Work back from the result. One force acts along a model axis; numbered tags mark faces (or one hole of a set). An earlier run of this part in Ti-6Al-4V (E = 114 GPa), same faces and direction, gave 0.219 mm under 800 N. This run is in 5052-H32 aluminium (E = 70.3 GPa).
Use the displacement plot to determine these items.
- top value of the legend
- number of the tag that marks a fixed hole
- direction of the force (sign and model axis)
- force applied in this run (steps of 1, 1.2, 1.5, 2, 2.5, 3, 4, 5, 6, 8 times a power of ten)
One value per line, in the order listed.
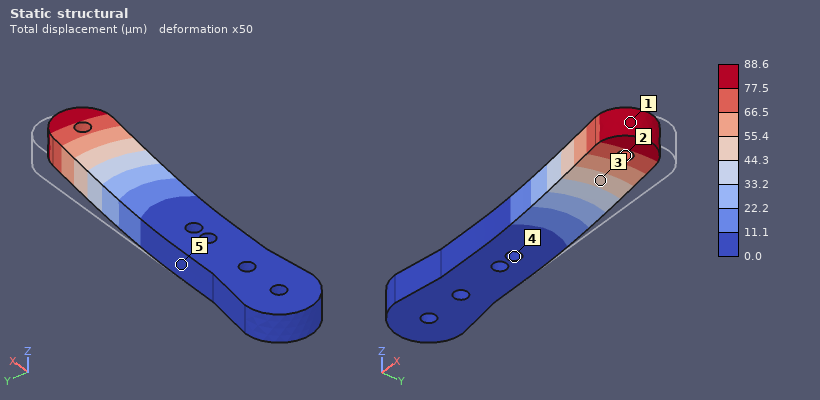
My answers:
88.6 µm
4
-Y
200 N
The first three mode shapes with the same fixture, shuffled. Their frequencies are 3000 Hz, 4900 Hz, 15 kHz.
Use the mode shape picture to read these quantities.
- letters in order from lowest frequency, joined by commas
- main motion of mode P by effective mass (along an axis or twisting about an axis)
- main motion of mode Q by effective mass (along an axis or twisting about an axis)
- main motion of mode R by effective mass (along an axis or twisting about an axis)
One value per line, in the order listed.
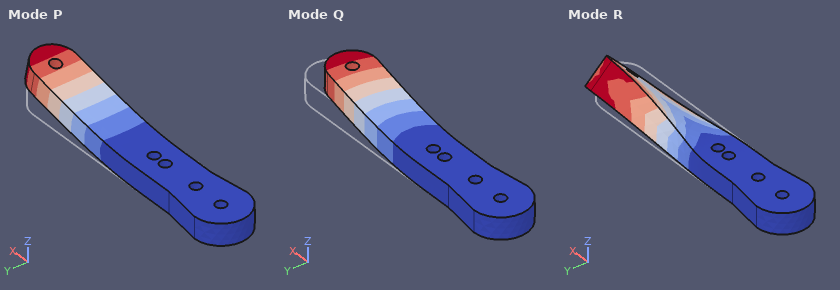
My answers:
P, Q, R
along Z
along Y
twisting about X
